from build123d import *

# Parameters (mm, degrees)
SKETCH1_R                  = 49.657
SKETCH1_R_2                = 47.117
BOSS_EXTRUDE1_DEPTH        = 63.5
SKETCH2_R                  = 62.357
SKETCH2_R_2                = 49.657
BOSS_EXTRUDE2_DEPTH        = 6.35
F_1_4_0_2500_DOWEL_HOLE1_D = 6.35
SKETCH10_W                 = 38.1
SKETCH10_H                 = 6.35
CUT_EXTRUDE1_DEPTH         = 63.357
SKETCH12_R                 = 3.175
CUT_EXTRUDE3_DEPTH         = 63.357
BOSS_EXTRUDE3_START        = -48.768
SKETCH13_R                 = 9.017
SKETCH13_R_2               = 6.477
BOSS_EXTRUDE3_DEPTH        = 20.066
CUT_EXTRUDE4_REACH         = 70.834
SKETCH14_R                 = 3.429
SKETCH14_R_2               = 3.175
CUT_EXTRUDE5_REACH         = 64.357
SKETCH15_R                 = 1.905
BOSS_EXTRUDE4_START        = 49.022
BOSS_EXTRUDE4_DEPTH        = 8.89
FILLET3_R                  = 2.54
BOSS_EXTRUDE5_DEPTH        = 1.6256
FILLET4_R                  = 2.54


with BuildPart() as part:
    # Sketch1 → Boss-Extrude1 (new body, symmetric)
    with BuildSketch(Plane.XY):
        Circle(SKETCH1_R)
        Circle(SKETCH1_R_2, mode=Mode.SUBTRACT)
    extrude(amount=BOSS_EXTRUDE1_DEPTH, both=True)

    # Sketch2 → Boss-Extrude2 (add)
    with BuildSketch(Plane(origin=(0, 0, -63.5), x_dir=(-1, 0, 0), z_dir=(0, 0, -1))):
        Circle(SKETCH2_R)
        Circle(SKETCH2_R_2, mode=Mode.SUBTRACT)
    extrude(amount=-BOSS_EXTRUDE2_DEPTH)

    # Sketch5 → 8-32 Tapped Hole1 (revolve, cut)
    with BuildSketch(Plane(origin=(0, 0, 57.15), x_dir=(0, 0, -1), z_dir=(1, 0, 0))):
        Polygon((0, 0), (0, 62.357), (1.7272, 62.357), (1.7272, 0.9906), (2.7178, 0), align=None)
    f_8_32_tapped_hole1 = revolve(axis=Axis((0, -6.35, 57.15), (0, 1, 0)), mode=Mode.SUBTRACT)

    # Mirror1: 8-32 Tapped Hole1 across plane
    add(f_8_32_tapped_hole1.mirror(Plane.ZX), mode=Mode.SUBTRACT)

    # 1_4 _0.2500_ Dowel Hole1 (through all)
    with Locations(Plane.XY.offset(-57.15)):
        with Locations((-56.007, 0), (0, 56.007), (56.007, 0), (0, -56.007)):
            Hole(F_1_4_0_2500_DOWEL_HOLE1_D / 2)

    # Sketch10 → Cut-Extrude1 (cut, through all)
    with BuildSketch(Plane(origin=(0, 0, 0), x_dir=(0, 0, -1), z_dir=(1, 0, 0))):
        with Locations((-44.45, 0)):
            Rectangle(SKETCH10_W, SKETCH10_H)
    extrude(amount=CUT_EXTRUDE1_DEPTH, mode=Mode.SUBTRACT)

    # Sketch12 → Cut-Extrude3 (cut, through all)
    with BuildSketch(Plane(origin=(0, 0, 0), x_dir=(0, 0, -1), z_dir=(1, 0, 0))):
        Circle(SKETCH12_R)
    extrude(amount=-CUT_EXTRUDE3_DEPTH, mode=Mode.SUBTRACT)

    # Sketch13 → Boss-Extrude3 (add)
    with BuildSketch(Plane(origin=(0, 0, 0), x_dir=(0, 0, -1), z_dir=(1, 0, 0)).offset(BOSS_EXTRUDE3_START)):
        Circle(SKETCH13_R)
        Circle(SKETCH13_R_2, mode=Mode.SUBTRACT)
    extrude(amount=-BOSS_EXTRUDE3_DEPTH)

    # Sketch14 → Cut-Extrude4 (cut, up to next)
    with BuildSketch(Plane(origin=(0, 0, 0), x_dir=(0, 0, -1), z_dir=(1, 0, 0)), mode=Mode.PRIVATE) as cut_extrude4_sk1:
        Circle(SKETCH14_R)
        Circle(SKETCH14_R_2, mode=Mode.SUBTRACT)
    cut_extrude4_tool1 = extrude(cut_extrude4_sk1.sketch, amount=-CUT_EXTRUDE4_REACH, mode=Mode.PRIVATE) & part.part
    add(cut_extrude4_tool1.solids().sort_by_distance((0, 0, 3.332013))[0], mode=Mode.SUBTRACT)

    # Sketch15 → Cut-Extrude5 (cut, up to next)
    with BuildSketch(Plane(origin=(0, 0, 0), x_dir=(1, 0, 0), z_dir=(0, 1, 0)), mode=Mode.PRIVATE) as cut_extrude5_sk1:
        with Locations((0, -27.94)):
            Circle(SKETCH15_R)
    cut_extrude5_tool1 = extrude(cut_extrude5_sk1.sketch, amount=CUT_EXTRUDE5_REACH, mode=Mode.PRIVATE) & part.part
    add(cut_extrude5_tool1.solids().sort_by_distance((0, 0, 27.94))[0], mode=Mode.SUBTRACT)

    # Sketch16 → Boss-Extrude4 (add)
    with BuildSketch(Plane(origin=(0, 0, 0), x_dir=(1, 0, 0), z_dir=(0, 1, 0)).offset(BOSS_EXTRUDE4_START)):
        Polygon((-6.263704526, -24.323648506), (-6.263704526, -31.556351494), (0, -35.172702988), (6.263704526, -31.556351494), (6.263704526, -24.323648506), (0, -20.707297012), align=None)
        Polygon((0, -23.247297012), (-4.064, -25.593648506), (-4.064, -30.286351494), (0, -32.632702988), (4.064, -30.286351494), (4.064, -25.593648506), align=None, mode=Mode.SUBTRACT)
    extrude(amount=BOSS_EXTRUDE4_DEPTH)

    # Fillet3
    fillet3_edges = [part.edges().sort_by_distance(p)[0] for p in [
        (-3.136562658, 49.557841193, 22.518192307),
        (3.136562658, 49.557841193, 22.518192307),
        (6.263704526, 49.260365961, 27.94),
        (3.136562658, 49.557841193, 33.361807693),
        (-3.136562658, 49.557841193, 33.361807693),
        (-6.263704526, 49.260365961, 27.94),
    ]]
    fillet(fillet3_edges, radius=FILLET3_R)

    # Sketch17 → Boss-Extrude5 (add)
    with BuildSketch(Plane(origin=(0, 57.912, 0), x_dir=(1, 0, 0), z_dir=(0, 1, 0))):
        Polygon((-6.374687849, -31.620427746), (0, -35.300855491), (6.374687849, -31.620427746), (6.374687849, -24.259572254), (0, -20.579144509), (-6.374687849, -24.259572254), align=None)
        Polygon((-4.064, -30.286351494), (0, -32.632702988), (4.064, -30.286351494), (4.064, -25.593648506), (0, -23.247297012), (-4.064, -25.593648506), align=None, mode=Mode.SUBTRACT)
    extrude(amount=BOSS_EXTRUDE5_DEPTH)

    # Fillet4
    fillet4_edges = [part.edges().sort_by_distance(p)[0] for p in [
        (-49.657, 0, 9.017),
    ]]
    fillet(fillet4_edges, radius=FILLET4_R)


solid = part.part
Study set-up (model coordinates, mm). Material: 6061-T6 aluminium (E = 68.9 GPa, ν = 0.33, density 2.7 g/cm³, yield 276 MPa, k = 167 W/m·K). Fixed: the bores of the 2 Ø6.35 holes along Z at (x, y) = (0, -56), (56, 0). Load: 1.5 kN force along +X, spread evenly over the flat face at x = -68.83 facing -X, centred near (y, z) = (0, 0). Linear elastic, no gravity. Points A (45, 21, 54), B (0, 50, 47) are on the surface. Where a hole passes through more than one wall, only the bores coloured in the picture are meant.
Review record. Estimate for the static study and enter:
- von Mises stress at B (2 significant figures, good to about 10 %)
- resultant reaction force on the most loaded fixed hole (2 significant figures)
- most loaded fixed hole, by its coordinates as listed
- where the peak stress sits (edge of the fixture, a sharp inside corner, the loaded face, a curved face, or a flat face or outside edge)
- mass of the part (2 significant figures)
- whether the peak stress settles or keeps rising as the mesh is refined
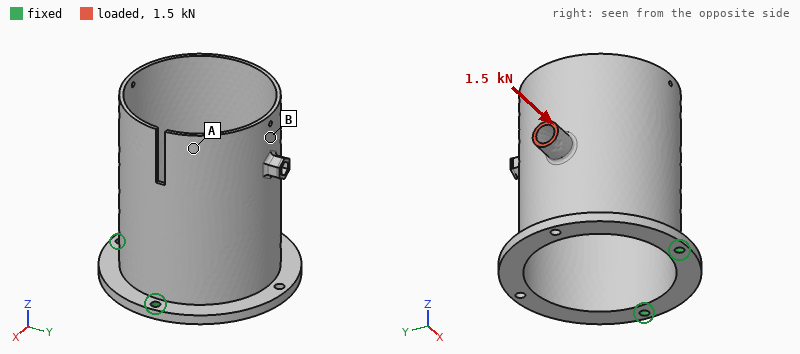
41 MPa
1.3 kN
(56, 0)
edge of the fixture
350 g
keeps rising
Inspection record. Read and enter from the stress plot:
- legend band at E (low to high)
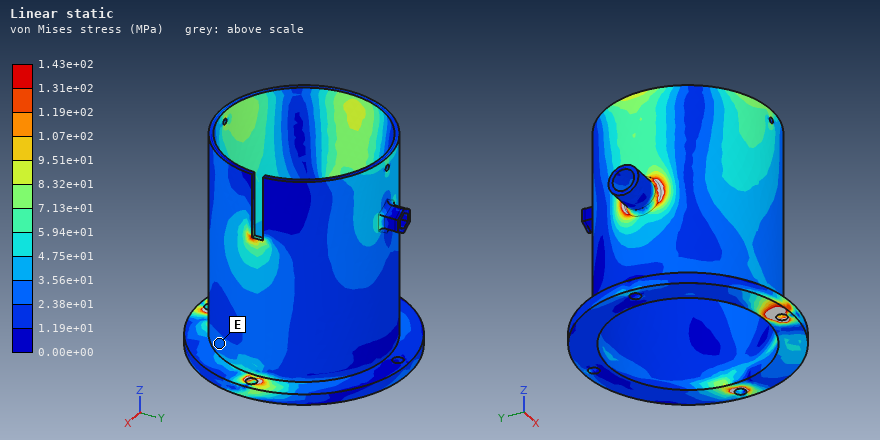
2.38e+01 to 3.56e+01 MPa
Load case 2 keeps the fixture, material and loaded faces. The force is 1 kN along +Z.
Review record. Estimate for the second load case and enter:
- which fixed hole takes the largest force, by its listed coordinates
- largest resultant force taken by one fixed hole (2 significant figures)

(0, -56)
1.1 kN
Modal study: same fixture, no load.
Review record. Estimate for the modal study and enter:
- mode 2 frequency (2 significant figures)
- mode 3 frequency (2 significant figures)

640 Hz
830 Hz
